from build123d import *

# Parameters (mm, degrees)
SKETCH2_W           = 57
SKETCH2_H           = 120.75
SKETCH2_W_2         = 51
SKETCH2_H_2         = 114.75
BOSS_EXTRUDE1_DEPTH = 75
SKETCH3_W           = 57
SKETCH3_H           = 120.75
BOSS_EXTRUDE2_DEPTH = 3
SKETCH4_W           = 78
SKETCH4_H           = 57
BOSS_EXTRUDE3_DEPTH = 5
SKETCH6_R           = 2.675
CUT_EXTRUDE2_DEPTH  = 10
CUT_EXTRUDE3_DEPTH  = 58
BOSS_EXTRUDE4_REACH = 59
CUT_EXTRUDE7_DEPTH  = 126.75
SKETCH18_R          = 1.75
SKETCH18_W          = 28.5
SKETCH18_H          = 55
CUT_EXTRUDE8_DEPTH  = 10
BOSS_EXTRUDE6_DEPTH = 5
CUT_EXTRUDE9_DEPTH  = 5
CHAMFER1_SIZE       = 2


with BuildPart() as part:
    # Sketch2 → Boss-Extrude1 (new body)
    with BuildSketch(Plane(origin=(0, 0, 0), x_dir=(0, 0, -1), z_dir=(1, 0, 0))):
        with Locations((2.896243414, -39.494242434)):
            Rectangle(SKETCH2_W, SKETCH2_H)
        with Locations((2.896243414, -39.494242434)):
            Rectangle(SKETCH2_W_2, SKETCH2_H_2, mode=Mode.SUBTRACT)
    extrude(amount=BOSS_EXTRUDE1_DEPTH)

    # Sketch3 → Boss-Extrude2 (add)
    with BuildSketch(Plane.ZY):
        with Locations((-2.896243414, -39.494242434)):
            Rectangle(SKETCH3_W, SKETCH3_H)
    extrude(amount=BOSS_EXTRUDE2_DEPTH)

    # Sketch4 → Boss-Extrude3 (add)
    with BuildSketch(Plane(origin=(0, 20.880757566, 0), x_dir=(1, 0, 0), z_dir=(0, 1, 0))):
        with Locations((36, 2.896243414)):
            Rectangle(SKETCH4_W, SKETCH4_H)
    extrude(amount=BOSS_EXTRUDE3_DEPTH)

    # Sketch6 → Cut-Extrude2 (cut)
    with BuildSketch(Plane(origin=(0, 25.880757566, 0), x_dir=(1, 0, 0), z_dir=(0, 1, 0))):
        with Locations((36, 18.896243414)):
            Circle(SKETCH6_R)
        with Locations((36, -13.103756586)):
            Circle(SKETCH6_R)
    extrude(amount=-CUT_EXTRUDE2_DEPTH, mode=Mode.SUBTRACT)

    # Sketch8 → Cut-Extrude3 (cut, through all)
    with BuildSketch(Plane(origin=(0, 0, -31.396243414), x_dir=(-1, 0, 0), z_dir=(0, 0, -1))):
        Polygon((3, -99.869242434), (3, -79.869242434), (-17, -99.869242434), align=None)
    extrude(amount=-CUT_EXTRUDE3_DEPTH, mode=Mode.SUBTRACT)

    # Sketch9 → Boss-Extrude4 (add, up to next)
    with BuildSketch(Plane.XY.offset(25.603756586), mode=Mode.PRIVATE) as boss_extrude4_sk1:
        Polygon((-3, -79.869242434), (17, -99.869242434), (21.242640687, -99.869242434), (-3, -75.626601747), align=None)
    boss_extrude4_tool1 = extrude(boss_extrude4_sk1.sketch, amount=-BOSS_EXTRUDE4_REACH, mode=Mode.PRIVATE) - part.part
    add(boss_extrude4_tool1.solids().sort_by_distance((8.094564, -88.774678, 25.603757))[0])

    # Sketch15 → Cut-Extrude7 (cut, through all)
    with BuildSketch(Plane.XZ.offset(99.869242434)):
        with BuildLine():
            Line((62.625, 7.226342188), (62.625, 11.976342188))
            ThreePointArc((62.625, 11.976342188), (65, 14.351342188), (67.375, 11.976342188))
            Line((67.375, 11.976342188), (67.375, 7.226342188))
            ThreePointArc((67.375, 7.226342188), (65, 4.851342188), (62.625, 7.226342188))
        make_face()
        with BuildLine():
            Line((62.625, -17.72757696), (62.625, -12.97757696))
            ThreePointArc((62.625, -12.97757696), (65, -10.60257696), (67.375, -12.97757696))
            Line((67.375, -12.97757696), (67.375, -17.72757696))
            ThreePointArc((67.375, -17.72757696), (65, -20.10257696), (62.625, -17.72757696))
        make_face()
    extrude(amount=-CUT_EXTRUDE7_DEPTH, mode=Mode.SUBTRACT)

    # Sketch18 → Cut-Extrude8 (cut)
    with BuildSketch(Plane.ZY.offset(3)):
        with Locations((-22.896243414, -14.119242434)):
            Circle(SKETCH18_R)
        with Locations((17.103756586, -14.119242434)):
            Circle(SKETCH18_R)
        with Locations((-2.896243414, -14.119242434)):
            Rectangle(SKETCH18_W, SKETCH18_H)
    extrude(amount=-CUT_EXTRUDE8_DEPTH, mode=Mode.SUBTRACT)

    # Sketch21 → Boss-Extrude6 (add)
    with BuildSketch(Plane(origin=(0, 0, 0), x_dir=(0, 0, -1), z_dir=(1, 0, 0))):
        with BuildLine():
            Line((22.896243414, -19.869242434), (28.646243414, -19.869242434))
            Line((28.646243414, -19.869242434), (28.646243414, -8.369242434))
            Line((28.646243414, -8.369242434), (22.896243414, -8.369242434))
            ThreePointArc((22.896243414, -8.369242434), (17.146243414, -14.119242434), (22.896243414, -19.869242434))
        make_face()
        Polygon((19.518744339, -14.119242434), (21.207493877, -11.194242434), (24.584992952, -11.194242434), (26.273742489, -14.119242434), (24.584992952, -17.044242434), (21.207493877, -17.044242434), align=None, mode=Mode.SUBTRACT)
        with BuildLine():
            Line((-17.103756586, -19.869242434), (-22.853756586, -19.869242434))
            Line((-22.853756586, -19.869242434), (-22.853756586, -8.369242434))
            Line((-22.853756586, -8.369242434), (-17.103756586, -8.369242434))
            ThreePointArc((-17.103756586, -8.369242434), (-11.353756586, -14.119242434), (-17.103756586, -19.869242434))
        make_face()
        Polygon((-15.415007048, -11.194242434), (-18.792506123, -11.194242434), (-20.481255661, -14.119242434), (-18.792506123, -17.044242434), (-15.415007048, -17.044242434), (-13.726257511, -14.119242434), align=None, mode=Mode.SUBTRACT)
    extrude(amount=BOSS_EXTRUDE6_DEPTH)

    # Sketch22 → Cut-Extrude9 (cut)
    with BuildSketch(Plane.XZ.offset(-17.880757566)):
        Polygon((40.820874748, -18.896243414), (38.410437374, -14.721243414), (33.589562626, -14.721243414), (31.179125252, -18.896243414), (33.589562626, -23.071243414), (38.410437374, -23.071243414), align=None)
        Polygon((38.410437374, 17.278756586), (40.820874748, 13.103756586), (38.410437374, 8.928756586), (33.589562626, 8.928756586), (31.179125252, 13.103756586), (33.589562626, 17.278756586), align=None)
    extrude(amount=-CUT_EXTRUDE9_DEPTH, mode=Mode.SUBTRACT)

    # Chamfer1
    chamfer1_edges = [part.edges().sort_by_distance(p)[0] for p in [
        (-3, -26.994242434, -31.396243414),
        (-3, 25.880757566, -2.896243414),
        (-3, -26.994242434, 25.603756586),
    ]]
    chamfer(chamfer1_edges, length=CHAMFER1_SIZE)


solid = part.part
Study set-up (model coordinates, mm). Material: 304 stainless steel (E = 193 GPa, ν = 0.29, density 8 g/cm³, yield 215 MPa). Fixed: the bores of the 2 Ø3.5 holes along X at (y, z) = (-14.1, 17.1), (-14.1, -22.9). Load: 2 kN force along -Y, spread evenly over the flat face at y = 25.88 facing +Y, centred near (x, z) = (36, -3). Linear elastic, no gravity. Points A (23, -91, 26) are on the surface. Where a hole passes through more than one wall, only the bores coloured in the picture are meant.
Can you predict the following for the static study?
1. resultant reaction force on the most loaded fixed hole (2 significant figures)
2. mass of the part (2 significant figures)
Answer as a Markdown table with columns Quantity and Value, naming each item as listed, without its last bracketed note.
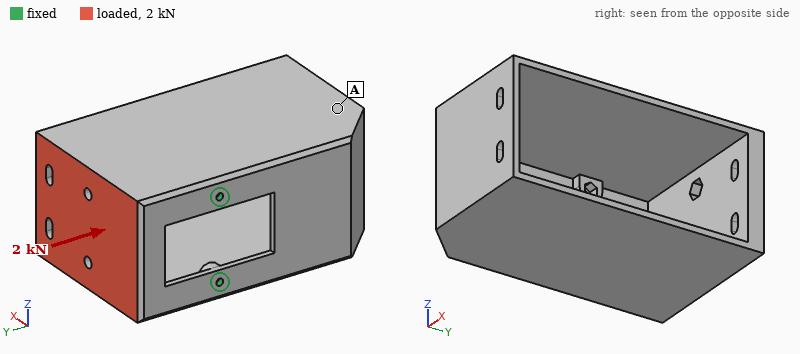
| Quantity | Value |
|---|---|
| resultant reaction force on the most loaded fixed hole | 1.0 kN |
| mass of the part | 890 g |
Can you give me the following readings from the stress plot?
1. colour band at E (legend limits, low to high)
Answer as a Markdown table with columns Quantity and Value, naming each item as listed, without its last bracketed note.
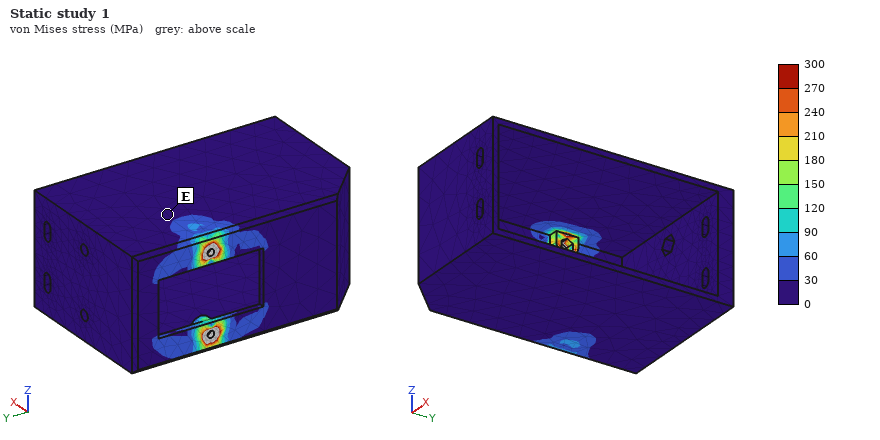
| Quantity | Value |
|---|---|
| colour band at E | 0 to 30 MPa |
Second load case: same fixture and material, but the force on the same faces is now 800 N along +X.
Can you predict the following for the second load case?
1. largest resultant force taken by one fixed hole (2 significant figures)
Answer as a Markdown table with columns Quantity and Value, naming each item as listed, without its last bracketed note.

| Quantity | Value |
|---|---|
| largest resultant force taken by one fixed hole | 400 N |
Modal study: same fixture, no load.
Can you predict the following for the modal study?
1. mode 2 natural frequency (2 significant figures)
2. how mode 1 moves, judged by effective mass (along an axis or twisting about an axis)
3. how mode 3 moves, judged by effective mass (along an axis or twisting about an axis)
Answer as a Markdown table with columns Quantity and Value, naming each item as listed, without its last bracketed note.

| Quantity | Value |
|---|---|
| mode 2 natural frequency | 690 Hz |
| how mode 1 moves, judged by effective mass | along Y |
| how mode 3 moves, judged by effective mass | along Z |
